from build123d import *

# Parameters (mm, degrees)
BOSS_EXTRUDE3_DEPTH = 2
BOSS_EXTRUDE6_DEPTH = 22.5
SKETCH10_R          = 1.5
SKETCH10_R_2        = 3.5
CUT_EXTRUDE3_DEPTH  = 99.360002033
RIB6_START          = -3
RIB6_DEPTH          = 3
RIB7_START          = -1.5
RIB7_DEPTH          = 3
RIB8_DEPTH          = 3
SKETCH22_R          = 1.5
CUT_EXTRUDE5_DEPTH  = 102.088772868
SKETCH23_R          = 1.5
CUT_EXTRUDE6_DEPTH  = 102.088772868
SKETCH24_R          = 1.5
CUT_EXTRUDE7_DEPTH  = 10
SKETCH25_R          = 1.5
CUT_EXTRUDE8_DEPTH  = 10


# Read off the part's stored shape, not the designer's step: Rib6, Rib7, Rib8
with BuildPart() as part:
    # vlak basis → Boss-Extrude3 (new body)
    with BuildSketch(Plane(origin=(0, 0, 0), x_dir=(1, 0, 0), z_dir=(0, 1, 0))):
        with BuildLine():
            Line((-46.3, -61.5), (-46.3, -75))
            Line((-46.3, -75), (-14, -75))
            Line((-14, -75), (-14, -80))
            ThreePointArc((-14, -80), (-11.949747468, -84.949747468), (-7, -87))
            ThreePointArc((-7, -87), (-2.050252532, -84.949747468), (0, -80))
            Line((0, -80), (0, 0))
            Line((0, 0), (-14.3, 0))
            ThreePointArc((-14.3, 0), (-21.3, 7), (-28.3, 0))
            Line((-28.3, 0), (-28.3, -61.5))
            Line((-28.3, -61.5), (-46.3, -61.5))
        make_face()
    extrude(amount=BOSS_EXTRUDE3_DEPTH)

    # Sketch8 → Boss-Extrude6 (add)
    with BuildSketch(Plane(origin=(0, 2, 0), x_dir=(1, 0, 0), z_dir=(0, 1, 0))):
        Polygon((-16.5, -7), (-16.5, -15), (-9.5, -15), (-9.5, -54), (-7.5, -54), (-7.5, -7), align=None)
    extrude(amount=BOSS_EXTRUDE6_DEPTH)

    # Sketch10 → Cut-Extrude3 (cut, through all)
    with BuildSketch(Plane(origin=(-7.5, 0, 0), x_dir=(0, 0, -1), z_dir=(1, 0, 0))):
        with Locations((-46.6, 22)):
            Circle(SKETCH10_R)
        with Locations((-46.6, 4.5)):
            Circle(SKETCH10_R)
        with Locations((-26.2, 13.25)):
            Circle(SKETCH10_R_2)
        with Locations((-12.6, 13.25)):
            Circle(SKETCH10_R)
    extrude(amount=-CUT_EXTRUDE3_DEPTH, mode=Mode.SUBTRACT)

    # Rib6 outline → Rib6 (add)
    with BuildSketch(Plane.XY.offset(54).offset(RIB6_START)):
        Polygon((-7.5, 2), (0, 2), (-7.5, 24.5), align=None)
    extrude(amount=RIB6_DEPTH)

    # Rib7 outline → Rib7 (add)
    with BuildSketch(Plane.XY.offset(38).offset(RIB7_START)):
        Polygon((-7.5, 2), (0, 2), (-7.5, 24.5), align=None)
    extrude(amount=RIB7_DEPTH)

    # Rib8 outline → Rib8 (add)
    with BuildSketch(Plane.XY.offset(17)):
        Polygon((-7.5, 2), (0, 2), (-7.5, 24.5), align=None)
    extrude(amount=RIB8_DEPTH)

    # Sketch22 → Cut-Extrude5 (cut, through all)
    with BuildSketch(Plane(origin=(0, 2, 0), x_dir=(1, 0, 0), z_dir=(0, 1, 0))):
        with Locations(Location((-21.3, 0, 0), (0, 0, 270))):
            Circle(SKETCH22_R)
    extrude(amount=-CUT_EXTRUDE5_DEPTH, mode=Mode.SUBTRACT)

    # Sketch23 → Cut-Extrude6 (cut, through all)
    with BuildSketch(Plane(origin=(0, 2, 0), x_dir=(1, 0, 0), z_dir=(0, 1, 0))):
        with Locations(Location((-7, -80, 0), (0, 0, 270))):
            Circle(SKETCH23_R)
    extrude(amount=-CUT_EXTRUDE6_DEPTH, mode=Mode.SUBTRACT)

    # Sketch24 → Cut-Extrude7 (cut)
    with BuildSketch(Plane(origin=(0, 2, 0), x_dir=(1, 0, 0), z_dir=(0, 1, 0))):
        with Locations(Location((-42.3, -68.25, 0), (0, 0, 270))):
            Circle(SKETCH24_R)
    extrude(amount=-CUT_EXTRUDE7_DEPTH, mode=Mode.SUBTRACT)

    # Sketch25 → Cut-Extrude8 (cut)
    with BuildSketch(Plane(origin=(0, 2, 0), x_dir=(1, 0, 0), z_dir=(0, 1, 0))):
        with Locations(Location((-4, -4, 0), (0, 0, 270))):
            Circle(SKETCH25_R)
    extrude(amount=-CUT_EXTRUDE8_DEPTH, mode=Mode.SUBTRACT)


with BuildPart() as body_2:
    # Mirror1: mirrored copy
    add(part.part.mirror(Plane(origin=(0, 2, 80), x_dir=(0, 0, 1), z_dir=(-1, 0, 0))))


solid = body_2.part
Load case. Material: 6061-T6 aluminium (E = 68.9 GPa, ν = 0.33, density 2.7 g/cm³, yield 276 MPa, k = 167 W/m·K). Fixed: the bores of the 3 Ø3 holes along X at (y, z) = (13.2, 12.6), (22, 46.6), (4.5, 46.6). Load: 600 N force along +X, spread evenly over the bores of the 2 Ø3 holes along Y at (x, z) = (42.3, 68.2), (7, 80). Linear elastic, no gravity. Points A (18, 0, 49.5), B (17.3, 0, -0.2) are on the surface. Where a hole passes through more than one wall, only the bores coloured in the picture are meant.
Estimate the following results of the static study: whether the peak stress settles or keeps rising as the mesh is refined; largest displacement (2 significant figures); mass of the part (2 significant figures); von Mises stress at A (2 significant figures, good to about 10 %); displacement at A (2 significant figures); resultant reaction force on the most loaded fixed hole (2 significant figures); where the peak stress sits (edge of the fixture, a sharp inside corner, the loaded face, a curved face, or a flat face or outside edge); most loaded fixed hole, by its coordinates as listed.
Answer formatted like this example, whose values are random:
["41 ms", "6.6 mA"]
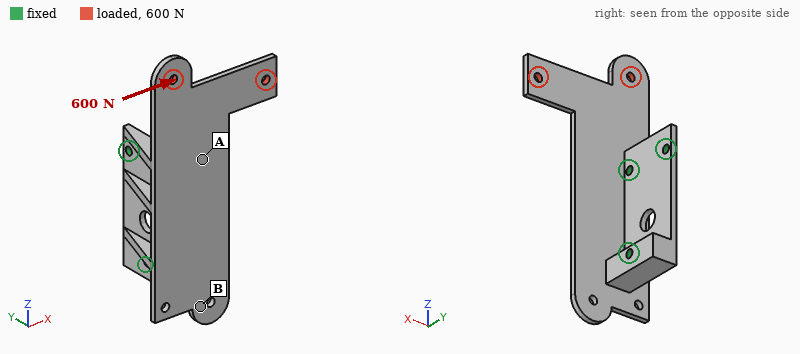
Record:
["keeps rising", "0.16 mm", "25 g", "30 MPa", "0.033 mm", "1.1 kN", "edge of the fixture", "(4.5, 46.6)"]
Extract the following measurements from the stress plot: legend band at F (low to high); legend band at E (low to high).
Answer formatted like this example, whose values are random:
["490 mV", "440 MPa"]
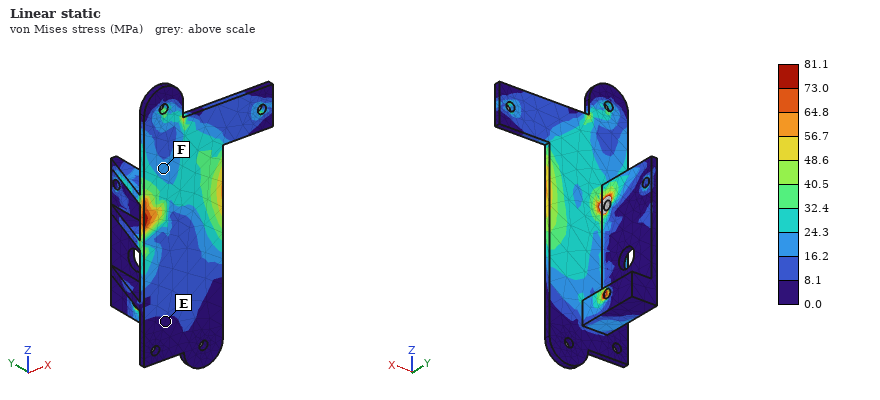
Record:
["16.2 to 24.3 MPa", "0.0 to 8.1 MPa"]
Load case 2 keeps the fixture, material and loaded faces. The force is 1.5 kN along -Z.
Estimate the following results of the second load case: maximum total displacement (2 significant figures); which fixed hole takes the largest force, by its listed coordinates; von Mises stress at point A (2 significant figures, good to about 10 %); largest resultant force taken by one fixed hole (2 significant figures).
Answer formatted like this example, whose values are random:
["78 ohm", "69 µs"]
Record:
["0.27 mm", "(4.5, 46.6)", "43 MPa", "1.2 kN"]
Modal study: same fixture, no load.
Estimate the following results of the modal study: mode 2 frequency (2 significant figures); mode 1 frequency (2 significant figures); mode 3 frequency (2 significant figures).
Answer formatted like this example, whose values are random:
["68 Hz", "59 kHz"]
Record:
["1900 Hz", "1200 Hz", "5000 Hz"]
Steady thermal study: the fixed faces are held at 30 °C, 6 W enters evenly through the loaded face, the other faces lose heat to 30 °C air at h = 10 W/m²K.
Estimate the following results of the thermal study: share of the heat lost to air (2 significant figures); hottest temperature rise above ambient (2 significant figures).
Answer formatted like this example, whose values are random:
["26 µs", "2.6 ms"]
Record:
["7.7 %", "29 K"]
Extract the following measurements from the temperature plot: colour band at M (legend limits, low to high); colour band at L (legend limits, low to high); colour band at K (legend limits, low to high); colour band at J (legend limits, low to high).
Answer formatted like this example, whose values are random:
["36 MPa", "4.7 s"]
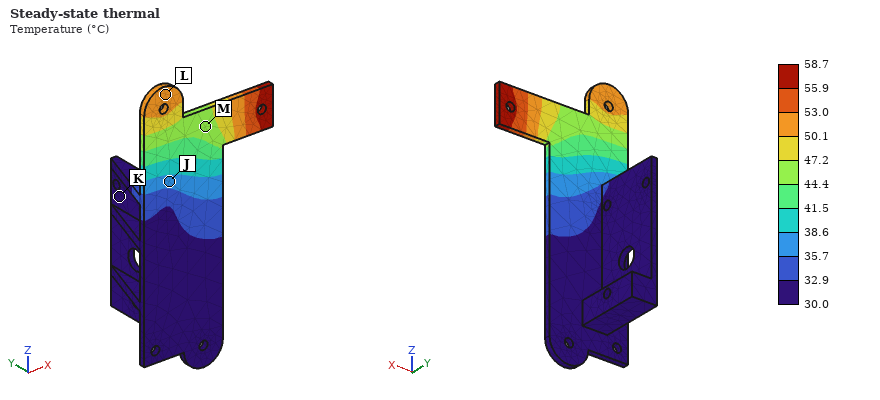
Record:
["44.4 to 47.2 °C", "50.1 to 53.0 °C", "30.0 to 32.9 °C", "35.7 to 38.6 °C"]
